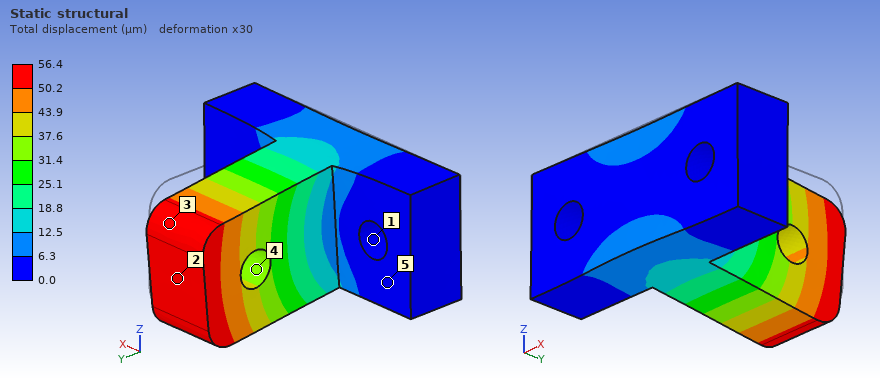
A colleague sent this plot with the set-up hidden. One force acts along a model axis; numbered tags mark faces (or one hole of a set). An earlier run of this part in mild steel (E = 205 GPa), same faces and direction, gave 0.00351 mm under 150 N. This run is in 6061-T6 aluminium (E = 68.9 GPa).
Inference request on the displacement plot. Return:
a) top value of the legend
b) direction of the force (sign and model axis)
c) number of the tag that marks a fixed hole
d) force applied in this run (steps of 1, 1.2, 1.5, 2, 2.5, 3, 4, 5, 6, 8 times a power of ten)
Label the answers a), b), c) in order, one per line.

a) 56.4 µm
b) -Z
c) 1
d) 800 N
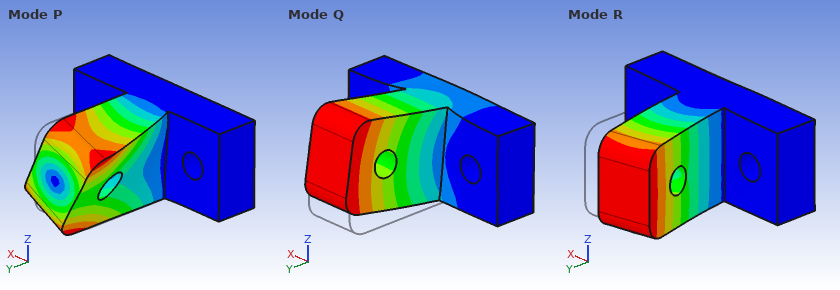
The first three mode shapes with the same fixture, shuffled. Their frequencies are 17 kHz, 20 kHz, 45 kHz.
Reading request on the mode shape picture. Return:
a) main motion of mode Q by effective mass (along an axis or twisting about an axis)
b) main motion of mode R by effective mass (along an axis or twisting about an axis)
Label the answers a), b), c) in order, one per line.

a) along Z
b) along X
